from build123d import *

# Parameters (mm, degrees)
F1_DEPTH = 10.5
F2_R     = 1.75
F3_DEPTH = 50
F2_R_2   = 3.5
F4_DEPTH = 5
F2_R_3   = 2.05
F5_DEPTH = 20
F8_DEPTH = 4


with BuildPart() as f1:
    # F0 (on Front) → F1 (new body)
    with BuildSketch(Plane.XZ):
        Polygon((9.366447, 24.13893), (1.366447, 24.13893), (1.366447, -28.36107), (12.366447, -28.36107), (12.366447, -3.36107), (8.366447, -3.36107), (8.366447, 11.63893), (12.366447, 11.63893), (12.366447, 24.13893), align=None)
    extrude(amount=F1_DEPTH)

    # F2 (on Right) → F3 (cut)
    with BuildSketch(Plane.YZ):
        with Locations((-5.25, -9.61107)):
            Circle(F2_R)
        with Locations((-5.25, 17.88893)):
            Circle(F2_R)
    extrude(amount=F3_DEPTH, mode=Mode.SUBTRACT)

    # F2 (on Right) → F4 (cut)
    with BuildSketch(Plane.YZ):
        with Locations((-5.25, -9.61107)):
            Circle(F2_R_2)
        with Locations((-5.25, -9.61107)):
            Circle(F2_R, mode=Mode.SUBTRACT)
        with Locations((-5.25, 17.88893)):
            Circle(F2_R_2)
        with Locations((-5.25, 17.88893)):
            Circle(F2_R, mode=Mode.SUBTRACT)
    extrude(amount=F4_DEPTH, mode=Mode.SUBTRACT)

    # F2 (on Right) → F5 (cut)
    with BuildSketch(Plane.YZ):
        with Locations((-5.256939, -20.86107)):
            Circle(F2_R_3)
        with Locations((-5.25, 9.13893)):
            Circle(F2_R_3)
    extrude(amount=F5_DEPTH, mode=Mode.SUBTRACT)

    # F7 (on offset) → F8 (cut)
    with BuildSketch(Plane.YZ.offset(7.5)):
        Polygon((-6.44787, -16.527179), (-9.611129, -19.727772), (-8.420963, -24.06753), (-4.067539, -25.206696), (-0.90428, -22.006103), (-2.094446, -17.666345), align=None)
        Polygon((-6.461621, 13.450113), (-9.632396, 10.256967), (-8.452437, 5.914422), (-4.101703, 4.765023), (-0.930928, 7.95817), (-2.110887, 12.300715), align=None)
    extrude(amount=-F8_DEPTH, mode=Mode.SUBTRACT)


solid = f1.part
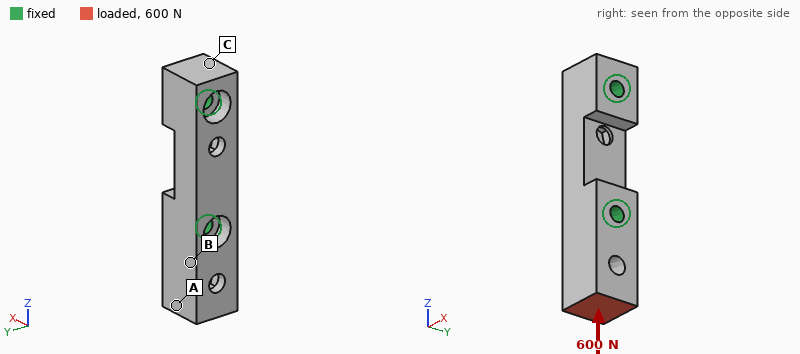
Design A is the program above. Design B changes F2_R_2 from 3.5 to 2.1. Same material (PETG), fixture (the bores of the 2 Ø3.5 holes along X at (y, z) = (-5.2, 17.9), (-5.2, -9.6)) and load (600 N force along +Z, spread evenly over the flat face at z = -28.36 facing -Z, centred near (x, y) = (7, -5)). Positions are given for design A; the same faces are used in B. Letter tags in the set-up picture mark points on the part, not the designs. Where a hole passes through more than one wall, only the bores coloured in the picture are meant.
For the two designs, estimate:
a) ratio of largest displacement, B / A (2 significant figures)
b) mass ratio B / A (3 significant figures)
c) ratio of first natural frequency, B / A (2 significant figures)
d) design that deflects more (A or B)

0.85
1.04
1.0
A
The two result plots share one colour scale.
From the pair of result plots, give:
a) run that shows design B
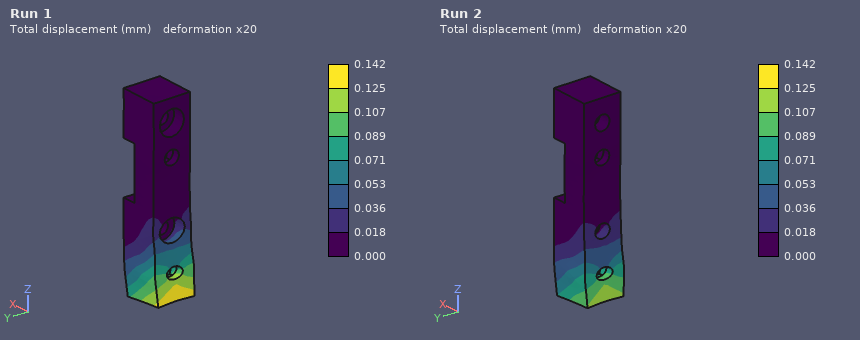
Run 2
